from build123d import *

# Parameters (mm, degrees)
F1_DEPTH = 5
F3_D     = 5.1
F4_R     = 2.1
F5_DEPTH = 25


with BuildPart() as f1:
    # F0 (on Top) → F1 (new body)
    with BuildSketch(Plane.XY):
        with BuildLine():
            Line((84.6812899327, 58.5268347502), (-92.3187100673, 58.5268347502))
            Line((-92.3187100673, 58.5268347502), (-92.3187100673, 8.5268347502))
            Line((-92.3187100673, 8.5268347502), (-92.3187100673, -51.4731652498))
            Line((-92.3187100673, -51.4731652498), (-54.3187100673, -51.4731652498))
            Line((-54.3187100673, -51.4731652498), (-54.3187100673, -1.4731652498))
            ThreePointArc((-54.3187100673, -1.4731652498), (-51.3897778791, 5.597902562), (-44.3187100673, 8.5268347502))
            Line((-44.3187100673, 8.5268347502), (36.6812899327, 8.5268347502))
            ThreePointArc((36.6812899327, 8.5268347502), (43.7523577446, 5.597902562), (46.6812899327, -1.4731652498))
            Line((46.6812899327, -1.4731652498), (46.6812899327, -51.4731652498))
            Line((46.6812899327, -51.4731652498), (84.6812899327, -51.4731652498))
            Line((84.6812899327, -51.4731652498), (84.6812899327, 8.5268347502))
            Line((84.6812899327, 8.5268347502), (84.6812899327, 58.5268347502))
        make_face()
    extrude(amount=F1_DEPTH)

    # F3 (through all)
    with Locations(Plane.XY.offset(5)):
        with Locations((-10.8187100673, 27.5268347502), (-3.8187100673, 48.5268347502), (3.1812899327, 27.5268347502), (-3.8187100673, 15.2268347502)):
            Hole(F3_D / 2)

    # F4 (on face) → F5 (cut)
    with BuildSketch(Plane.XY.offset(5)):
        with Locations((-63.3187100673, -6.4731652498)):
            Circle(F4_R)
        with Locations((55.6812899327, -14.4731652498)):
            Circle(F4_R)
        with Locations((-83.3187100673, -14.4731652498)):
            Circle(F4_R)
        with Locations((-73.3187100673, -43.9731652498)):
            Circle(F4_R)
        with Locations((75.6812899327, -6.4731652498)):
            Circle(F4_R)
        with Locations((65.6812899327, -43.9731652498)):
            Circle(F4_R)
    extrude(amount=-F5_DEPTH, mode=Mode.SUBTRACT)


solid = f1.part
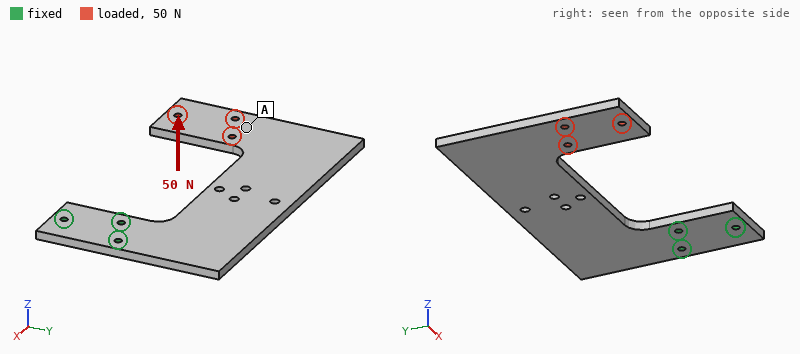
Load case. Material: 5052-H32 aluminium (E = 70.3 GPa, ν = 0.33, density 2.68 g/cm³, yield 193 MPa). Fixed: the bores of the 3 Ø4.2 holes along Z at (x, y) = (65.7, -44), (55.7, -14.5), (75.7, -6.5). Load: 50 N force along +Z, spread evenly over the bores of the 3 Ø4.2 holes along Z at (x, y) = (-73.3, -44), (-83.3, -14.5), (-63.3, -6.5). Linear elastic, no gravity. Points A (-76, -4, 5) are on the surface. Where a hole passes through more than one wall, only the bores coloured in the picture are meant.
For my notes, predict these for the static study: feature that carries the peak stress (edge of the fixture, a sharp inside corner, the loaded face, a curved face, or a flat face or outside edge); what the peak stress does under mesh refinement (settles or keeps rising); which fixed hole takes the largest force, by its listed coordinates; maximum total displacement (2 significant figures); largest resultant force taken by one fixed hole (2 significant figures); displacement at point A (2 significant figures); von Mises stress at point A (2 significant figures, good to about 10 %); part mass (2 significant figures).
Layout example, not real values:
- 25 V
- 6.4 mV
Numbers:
- edge of the fixture
- keeps rising
- (55.7, -14.5)
- 2.4 mm
- 290 N
- 1.8 mm
- 6.1 MPa
- 180 g
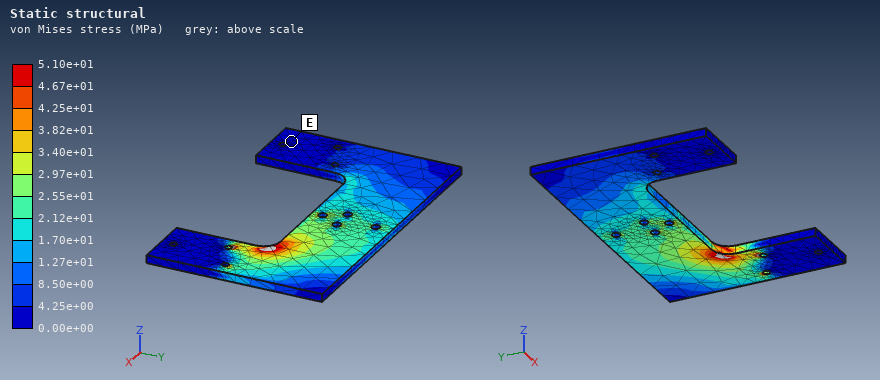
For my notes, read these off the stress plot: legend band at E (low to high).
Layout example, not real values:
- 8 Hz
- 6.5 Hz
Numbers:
- 0.00e+00 to 4.25e+00 MPa
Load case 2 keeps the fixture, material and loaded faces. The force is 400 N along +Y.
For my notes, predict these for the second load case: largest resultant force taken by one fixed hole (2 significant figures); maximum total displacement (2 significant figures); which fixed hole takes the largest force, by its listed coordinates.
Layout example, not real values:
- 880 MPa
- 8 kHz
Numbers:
- 2.1 kN
- 0.33 mm
- (55.7, -14.5)
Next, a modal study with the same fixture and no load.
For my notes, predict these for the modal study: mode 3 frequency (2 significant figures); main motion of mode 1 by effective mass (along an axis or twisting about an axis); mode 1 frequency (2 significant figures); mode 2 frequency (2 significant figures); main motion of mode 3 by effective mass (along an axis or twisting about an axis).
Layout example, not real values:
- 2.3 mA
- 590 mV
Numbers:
- 710 Hz
- along Z
- 110 Hz
- 280 Hz
- along Y
